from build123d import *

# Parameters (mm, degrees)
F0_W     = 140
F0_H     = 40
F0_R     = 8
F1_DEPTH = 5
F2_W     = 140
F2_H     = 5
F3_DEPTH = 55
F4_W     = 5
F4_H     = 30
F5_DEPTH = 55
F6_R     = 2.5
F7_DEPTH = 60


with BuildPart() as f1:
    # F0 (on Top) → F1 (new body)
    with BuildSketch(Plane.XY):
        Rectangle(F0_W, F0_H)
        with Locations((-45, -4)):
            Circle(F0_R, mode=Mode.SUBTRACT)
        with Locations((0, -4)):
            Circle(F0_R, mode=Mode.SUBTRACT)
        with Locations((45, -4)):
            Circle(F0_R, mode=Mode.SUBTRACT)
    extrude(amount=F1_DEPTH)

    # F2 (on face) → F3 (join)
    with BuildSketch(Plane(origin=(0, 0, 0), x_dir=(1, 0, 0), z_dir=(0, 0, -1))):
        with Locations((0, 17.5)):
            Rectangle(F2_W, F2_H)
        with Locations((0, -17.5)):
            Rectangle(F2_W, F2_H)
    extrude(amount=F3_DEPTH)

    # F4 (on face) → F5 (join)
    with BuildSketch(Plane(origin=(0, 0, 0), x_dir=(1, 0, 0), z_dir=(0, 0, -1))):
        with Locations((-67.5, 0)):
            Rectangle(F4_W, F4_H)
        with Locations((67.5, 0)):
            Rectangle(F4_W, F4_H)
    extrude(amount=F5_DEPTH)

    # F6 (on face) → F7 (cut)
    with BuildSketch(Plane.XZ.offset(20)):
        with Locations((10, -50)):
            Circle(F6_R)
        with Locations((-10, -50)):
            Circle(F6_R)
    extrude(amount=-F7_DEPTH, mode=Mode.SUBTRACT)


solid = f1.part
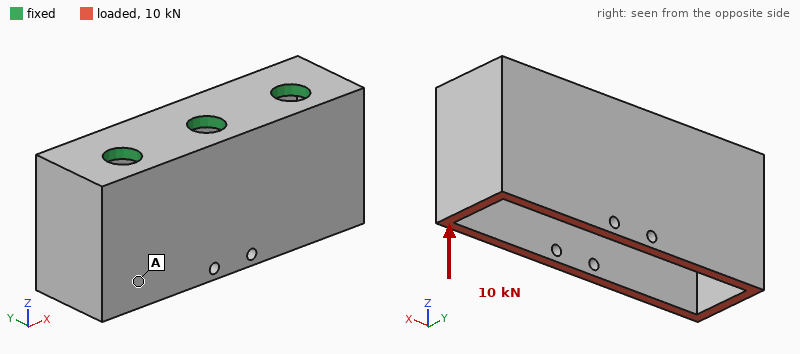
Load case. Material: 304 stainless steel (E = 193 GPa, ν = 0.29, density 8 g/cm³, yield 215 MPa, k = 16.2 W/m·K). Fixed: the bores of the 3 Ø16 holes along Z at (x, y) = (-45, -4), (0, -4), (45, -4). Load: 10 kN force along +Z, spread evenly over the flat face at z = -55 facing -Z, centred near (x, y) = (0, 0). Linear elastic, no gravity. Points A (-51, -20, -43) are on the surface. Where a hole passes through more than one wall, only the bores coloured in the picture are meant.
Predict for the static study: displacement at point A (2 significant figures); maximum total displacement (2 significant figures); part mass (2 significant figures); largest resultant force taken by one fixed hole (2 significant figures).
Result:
16 µm
55 µm
940 g
3.8 kN
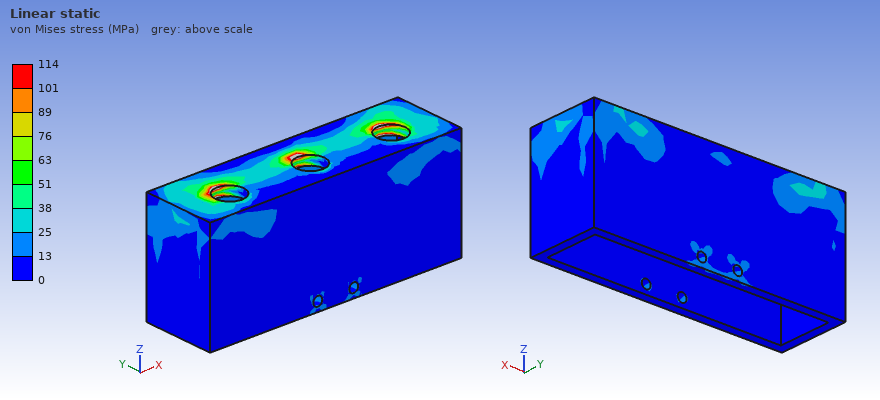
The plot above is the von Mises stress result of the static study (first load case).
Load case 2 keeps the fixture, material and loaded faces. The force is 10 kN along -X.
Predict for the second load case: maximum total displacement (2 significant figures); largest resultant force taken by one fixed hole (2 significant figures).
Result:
61 µm
6.3 kN
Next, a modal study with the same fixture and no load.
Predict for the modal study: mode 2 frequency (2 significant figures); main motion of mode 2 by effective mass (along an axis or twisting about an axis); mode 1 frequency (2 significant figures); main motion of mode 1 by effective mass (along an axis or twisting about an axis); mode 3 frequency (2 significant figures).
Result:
1800 Hz
twisting about Z
1400 Hz
along Y
1900 Hz
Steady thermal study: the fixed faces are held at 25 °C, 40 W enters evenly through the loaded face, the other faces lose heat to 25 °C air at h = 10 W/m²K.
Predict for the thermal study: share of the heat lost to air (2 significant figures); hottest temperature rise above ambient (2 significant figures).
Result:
44 %
81 K
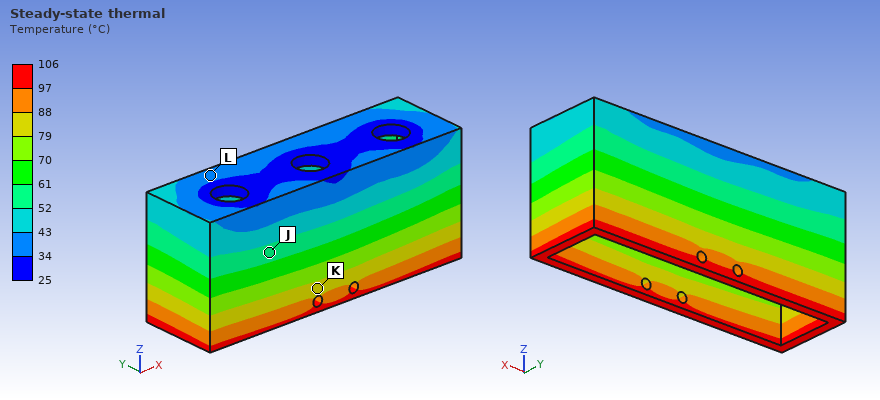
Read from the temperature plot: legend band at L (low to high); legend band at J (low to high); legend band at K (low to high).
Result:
34 to 43 °C
52 to 61 °C
79 to 88 °C
